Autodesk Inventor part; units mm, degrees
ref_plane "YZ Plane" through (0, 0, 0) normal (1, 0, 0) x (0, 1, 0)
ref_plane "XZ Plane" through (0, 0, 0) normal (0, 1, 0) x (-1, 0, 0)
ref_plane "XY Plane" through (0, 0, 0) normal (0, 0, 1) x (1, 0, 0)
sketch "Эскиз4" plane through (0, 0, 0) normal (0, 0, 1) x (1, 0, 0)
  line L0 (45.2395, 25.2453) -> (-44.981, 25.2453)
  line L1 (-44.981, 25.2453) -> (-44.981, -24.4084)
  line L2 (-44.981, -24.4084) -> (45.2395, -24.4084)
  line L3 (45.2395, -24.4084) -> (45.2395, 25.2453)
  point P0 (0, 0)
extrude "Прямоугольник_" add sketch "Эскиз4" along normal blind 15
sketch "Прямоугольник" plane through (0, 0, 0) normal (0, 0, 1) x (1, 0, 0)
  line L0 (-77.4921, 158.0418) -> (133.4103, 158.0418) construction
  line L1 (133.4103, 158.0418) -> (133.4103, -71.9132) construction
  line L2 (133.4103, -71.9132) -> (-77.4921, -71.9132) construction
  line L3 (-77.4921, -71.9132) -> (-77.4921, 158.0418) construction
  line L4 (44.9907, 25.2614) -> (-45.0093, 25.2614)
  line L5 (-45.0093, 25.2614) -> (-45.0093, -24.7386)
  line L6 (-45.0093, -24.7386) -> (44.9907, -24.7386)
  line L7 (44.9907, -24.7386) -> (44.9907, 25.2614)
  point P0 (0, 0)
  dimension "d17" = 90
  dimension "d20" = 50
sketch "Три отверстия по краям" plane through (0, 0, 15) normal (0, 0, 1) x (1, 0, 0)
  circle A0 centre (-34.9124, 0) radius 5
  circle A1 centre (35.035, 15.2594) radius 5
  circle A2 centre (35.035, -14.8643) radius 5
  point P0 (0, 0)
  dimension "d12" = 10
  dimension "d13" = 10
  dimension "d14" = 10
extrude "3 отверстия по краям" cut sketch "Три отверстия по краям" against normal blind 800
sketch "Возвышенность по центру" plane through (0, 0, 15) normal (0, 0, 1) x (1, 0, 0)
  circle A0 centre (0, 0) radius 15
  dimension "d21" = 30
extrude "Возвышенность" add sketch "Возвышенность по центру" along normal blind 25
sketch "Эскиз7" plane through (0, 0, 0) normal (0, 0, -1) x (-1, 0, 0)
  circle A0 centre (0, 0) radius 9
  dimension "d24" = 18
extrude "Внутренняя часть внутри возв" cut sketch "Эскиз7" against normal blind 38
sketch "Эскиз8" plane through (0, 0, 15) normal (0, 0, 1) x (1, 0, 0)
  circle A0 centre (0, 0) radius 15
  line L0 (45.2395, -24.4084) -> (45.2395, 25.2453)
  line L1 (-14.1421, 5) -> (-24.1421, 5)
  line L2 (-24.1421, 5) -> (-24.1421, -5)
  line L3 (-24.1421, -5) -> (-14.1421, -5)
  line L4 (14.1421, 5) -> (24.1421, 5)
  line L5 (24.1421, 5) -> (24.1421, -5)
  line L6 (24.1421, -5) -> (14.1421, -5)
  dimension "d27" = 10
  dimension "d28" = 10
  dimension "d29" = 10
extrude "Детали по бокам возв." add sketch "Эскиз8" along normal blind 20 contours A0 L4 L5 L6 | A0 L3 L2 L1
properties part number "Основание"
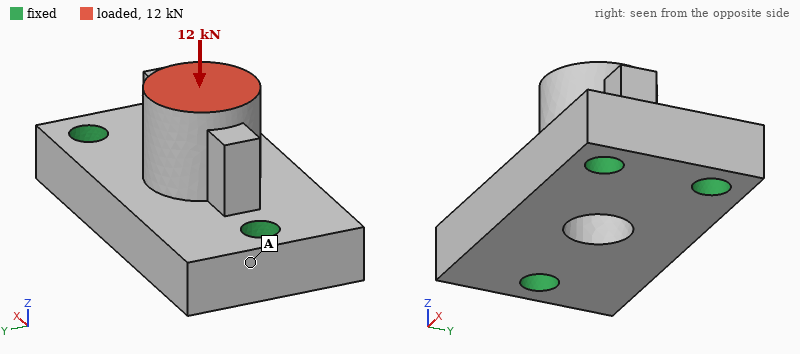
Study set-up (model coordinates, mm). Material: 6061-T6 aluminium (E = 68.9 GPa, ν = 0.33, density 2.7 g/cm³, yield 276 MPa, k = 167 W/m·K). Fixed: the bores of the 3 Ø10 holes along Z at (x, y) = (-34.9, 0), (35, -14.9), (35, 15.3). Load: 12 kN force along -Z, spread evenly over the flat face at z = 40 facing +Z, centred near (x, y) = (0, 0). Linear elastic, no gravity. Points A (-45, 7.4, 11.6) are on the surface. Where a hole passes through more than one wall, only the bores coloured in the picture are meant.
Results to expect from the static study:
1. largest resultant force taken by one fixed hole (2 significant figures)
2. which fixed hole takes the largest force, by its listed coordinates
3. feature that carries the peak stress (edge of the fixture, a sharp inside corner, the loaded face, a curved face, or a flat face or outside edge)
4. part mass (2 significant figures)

6.0 kN
(-34.9, 0)
the loaded face
200 g
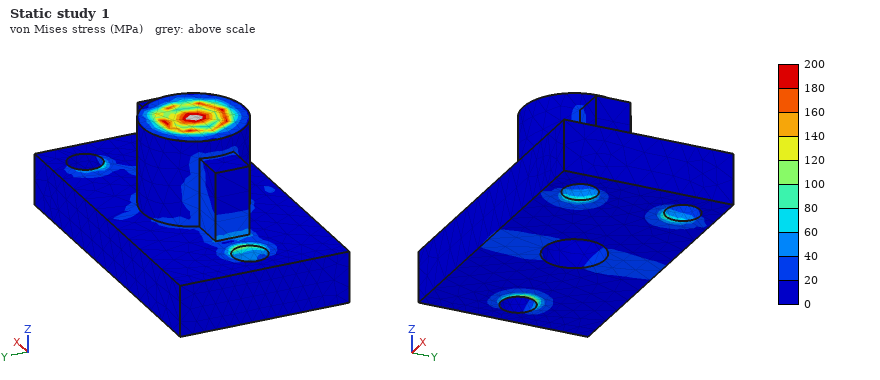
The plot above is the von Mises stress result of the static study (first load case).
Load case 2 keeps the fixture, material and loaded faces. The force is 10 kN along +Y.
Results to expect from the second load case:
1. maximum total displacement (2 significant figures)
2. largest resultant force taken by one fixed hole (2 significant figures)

0.17 mm
6.8 kN
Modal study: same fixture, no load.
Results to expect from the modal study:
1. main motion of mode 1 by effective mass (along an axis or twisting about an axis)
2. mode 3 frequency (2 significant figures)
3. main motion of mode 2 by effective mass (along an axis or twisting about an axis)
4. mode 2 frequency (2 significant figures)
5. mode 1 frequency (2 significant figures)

along Y
16 kHz
along Z
12 kHz
8700 Hz
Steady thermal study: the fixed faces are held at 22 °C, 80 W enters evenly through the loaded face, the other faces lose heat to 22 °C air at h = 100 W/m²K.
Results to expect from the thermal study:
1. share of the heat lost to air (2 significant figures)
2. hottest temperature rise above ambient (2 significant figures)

15 %
37 K
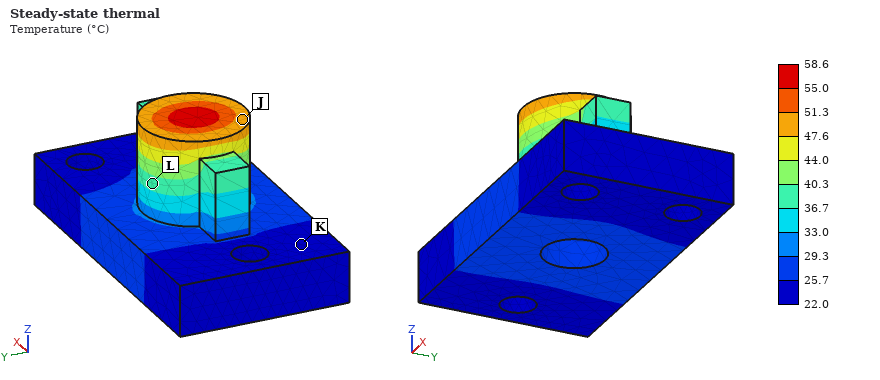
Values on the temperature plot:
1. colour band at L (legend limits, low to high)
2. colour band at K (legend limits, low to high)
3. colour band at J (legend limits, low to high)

36.7 to 40.3 °C
22.0 to 25.7 °C
47.6 to 51.3 °C
